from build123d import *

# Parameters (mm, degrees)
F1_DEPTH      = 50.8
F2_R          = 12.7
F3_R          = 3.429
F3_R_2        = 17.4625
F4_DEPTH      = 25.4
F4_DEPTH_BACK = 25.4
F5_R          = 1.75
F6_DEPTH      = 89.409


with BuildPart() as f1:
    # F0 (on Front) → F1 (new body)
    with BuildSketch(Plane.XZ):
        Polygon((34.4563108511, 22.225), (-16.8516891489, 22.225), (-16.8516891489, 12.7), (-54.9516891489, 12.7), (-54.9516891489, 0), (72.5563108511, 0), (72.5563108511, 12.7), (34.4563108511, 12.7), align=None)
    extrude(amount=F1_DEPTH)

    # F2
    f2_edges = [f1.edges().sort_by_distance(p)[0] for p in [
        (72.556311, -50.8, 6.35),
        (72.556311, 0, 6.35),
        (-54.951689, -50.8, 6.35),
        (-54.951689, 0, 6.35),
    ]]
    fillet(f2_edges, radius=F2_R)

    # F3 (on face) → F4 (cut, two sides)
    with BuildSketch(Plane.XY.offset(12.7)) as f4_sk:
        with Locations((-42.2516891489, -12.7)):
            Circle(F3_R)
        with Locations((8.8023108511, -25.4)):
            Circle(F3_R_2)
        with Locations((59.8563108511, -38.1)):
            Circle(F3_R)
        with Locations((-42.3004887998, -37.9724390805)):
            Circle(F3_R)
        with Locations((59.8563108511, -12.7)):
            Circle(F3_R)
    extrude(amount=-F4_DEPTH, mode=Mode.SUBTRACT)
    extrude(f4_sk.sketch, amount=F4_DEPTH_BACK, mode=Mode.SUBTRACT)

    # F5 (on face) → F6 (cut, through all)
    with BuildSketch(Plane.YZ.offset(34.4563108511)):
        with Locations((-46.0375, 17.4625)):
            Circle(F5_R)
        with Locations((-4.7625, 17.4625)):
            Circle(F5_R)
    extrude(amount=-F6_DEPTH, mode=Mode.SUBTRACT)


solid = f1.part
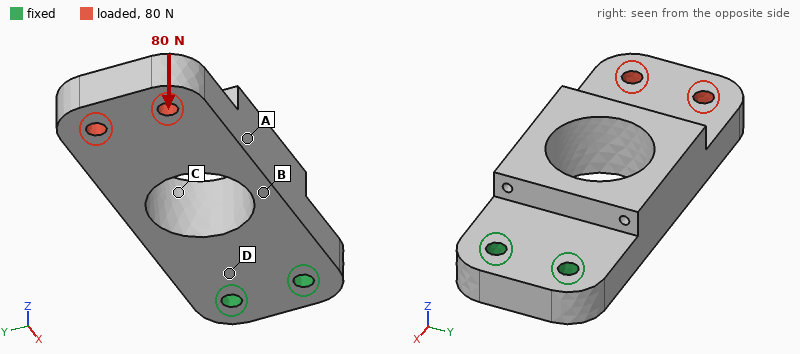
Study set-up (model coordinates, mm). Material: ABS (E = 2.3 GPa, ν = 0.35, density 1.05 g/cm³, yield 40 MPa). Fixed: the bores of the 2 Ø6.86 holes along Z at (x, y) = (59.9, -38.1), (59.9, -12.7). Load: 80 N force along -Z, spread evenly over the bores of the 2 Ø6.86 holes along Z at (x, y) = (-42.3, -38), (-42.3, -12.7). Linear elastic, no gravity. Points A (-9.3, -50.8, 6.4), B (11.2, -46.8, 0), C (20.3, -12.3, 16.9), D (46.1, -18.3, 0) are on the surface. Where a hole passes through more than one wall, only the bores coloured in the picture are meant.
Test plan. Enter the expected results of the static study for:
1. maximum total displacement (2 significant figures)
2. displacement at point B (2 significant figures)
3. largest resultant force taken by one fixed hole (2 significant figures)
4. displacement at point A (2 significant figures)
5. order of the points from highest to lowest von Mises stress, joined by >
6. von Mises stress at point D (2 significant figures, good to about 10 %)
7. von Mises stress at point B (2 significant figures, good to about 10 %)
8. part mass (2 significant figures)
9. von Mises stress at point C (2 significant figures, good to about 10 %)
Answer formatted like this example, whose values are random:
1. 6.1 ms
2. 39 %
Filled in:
1. 1.5 mm
2. 0.40 mm
3. 41 N
4. 0.68 mm
5. D > B > C > A
6. 4.5 MPa
7. 3.2 MPa
8. 85 g
9. 2.0 MPa
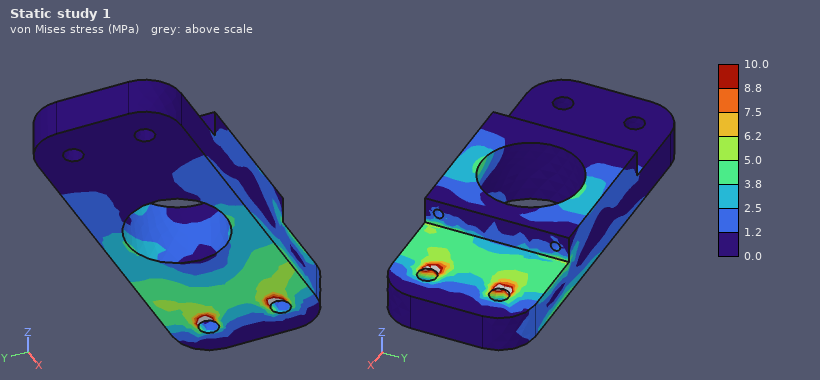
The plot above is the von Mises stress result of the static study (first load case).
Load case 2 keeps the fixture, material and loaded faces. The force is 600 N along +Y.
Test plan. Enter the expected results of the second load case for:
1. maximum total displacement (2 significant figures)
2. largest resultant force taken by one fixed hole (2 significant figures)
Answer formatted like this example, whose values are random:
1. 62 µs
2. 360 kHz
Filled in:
1. 1.4 mm
2. 2.1 kN
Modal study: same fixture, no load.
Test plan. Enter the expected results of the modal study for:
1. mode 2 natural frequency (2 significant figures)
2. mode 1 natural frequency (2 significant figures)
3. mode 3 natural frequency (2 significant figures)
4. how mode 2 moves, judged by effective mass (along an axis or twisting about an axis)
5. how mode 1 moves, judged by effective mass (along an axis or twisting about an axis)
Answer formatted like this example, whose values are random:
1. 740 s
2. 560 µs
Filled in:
1. 630 Hz
2. 250 Hz
3. 950 Hz
4. along Y
5. along Z
